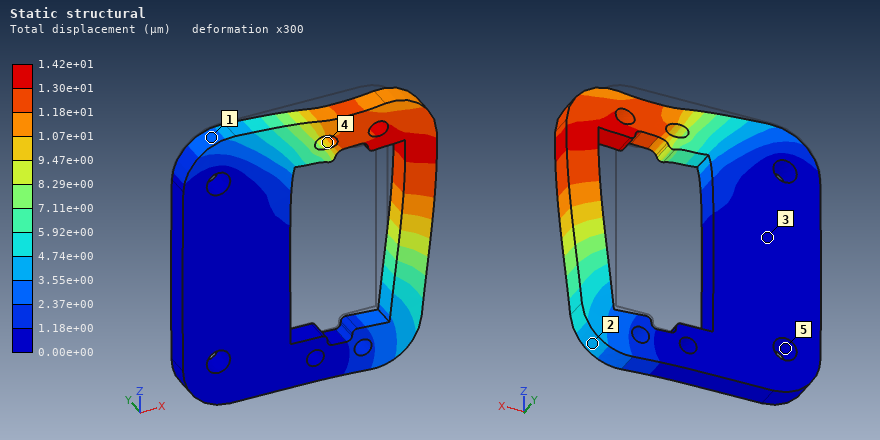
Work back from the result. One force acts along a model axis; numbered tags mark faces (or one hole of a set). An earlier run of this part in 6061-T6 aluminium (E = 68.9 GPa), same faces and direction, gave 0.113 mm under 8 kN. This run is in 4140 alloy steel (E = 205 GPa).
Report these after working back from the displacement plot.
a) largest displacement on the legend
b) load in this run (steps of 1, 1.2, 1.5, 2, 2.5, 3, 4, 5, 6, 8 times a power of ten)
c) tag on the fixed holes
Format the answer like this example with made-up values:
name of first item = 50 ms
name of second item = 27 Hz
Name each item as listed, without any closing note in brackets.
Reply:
largest displacement on the legend = 1.42e+01 µm
load in this run = 3 kN
tag on the fixed holes = 5
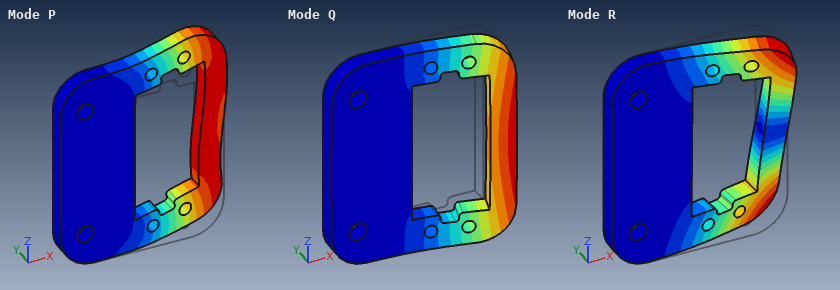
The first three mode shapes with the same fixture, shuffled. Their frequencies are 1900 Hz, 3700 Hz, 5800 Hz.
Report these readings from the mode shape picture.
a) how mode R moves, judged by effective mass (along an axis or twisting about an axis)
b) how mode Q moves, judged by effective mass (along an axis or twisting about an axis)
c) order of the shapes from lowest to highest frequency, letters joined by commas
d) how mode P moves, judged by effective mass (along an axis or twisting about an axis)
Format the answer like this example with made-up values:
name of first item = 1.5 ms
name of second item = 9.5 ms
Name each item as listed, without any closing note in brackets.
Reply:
how mode R moves, judged by effective mass = twisting about X
how mode Q moves, judged by effective mass = along Y
order of the shapes from lowest to highest frequency, letters joined by commas = Q, R, P
how mode P moves, judged by effective mass = along Z
